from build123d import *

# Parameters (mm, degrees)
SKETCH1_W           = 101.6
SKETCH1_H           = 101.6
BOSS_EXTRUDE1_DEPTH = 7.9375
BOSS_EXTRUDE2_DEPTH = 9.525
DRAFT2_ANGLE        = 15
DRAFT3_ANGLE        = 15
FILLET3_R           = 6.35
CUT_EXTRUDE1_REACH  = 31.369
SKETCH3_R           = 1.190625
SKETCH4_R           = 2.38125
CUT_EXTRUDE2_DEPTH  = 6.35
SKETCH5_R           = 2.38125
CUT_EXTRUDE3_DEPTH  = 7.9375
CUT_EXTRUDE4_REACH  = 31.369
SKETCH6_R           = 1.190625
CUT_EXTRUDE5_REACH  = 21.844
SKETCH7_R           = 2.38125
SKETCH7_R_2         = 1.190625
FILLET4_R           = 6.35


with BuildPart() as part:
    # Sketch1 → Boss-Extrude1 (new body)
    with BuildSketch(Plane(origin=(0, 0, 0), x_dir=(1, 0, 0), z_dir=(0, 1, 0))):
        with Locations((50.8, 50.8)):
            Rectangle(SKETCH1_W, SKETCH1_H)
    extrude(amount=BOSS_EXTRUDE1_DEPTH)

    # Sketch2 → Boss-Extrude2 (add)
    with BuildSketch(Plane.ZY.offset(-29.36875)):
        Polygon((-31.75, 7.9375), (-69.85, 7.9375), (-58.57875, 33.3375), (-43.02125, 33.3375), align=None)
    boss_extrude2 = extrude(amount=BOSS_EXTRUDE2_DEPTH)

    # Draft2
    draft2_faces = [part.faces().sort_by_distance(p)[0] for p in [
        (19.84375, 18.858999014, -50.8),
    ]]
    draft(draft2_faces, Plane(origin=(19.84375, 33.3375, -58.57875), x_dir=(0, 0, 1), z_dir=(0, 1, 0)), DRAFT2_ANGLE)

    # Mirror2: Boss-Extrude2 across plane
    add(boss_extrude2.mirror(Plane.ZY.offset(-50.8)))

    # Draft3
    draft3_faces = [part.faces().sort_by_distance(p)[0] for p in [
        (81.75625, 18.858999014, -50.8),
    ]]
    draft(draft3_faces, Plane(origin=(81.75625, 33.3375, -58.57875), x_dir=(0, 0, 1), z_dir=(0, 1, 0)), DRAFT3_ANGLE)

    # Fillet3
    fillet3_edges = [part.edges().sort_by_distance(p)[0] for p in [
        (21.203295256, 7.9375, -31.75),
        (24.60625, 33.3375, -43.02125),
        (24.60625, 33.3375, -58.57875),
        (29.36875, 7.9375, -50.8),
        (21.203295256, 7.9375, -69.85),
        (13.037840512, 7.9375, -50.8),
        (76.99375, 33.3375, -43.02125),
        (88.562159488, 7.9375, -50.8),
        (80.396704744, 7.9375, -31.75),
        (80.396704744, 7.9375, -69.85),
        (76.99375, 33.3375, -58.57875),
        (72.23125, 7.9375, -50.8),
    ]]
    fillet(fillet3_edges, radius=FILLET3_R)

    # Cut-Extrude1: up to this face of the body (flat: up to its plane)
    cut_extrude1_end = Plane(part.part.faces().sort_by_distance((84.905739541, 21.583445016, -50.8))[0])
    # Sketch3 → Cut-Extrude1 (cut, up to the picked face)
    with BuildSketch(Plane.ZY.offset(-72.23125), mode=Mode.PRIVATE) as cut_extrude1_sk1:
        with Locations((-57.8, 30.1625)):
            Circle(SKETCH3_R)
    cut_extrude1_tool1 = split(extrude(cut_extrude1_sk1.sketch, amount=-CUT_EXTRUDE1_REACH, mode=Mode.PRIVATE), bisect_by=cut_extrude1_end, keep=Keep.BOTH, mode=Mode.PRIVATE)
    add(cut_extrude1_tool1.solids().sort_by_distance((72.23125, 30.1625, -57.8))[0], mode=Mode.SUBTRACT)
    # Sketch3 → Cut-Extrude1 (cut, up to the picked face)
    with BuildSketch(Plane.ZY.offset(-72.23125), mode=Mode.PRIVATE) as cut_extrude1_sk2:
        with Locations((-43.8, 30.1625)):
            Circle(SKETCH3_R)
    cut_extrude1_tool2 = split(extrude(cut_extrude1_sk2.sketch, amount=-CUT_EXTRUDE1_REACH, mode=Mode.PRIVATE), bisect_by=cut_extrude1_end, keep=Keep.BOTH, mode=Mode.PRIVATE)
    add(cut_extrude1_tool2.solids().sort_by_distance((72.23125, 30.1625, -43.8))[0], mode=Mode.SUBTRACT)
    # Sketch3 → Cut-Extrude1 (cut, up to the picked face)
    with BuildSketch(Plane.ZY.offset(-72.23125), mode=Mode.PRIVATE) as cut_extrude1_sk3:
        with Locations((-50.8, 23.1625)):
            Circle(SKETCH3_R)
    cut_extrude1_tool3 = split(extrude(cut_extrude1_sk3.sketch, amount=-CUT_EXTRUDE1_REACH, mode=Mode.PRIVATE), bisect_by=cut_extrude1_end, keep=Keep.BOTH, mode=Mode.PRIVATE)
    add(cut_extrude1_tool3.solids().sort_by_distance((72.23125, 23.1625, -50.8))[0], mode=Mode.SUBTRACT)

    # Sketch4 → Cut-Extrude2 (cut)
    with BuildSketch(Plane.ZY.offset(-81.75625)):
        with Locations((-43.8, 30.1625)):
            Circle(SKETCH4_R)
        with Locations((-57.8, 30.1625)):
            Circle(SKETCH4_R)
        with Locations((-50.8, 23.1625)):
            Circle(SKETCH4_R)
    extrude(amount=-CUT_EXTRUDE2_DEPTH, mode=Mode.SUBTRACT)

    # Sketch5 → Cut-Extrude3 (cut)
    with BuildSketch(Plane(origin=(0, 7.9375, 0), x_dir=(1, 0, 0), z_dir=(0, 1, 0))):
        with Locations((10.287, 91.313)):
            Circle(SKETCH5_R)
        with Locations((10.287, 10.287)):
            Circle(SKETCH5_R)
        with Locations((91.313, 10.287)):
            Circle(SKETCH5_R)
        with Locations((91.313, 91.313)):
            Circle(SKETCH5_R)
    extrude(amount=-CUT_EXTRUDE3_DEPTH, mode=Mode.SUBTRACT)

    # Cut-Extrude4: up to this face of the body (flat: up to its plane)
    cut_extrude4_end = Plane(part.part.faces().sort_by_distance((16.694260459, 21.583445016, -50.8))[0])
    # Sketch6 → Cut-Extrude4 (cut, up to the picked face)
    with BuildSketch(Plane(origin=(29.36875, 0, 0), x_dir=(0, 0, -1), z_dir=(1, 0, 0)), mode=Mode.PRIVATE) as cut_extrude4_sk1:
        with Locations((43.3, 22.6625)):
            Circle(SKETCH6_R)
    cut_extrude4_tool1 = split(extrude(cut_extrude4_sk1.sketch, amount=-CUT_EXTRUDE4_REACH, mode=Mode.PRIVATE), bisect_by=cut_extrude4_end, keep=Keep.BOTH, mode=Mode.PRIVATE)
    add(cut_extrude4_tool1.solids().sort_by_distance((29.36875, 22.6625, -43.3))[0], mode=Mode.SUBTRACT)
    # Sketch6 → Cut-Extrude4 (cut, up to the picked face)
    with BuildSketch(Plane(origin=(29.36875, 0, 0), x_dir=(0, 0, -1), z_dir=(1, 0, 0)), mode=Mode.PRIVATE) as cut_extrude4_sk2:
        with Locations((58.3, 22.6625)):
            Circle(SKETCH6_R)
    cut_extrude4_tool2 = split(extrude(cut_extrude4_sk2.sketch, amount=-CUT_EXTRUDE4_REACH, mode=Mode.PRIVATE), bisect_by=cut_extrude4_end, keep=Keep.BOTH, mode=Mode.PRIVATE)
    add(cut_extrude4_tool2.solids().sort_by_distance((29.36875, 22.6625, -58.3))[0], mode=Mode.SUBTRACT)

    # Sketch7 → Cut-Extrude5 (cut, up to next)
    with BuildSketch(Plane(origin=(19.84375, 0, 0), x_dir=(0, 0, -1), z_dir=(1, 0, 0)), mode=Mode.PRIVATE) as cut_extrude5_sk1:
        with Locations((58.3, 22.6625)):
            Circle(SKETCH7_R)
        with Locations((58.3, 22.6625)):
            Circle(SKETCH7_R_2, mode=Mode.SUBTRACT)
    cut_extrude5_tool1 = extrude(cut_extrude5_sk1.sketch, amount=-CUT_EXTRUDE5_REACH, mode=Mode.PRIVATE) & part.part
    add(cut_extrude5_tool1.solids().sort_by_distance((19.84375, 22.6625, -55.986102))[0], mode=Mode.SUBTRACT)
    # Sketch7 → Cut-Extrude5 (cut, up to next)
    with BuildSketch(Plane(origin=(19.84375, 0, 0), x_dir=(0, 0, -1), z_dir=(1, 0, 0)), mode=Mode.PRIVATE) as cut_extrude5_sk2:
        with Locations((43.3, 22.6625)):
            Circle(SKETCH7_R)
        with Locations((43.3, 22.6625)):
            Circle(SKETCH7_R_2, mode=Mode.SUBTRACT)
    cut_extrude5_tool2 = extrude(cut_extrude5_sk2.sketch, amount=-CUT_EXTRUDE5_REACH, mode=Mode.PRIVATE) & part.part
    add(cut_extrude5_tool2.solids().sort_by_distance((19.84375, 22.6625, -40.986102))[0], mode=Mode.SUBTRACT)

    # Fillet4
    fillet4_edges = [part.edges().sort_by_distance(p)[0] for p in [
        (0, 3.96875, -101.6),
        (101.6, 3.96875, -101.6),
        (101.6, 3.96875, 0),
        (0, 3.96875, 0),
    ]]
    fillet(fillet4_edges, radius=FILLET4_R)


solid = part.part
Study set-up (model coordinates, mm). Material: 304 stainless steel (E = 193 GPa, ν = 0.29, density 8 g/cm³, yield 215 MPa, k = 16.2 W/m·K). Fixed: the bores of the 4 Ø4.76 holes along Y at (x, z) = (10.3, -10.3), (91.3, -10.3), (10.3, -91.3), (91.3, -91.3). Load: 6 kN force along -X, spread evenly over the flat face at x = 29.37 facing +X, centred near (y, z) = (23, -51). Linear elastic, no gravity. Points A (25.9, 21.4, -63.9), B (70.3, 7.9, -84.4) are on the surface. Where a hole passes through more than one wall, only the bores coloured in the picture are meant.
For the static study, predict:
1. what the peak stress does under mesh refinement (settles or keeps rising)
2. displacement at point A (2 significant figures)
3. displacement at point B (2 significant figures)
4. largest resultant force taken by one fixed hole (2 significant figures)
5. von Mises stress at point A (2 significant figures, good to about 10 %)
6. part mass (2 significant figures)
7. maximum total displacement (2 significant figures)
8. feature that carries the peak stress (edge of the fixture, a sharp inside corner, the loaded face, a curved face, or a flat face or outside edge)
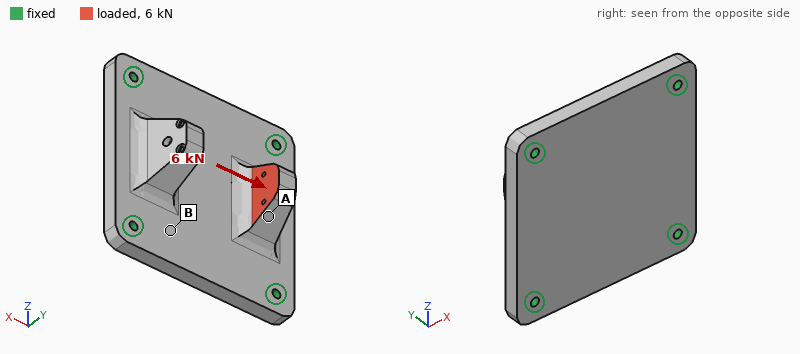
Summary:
keeps rising
33 µm
9.7 µm
2.0 kN
36 MPa
800 g
61 µm
edge of the fixture
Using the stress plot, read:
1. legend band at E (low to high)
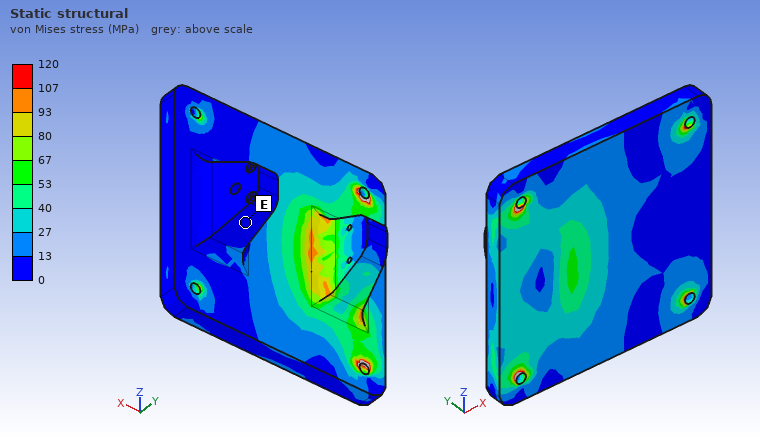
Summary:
0 to 13 MPa
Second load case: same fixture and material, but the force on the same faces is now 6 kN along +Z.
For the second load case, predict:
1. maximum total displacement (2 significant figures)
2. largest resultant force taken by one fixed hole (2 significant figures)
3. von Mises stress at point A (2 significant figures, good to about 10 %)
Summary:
22 µm
2.8 kN
37 MPa
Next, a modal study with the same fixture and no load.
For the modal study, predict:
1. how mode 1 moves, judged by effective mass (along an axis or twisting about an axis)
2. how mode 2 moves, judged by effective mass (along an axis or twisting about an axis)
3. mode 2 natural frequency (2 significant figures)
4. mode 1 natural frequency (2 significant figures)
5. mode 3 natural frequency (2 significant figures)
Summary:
along Y
twisting about Z
5800 Hz
3600 Hz
6300 Hz
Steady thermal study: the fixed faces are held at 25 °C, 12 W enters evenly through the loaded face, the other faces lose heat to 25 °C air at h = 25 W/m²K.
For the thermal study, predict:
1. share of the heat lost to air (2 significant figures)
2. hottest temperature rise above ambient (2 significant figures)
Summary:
49 %
56 K
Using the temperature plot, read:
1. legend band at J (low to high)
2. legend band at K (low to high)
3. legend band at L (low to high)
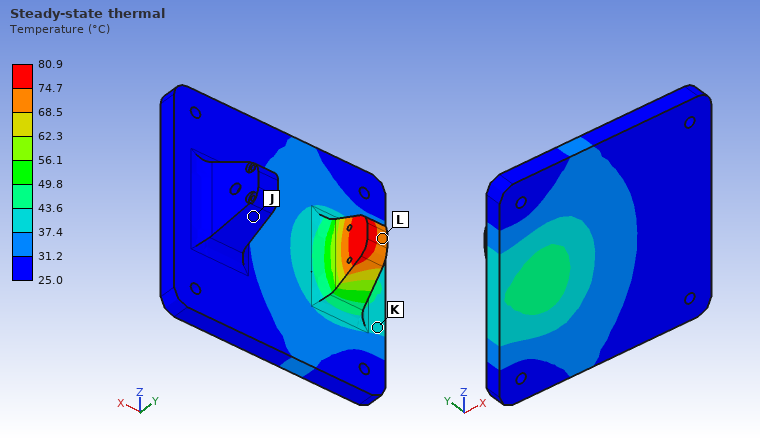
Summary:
25.0 to 31.2 °C
37.4 to 43.6 °C
68.5 to 74.7 °C
